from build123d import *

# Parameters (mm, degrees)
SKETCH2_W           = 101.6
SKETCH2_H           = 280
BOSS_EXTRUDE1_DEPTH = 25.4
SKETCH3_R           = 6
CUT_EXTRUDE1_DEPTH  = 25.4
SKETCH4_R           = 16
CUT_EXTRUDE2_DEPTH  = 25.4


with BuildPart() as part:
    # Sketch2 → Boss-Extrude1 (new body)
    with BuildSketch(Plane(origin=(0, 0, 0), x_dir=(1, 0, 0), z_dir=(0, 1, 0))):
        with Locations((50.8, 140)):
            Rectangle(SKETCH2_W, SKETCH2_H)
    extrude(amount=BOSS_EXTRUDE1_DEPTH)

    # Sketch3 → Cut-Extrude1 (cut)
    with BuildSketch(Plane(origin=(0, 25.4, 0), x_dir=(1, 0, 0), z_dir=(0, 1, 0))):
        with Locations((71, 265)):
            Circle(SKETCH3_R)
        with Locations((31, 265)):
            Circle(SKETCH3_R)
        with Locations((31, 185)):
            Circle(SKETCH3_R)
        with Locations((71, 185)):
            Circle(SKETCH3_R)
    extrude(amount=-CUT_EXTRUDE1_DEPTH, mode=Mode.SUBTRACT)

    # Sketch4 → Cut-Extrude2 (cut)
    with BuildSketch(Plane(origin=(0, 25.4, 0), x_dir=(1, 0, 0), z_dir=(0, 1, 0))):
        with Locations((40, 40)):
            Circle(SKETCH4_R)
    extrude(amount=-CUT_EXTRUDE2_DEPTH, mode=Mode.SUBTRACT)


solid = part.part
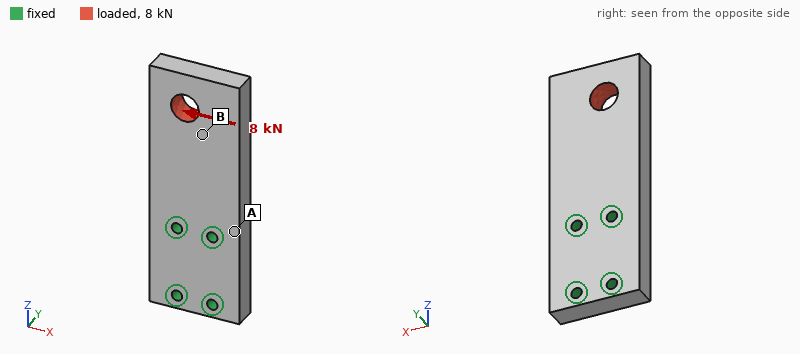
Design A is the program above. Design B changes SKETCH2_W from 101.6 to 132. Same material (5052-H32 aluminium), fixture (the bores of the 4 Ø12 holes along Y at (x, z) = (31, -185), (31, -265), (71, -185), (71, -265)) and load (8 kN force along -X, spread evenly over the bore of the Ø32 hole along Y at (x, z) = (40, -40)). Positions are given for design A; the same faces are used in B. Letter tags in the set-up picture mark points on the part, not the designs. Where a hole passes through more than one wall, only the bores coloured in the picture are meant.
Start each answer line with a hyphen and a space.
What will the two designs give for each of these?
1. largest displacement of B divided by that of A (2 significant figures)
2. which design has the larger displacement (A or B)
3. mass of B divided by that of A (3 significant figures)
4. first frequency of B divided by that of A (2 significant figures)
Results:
- 0.63
- A
- 1.31
- 0.97
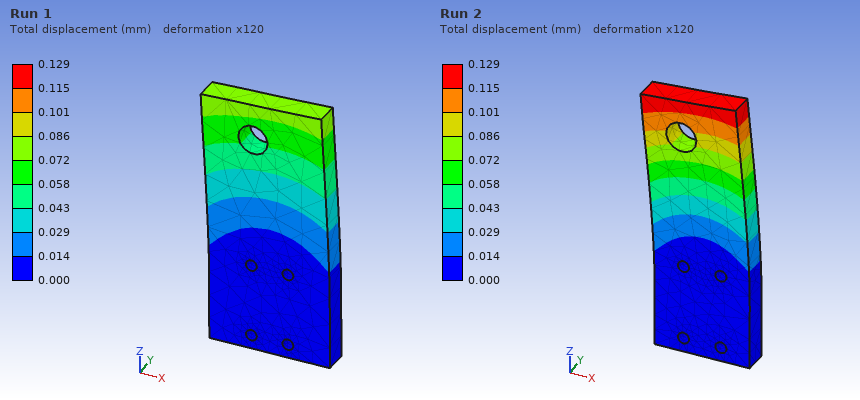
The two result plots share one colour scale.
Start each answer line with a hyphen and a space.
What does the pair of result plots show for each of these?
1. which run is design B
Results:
- Run 1
